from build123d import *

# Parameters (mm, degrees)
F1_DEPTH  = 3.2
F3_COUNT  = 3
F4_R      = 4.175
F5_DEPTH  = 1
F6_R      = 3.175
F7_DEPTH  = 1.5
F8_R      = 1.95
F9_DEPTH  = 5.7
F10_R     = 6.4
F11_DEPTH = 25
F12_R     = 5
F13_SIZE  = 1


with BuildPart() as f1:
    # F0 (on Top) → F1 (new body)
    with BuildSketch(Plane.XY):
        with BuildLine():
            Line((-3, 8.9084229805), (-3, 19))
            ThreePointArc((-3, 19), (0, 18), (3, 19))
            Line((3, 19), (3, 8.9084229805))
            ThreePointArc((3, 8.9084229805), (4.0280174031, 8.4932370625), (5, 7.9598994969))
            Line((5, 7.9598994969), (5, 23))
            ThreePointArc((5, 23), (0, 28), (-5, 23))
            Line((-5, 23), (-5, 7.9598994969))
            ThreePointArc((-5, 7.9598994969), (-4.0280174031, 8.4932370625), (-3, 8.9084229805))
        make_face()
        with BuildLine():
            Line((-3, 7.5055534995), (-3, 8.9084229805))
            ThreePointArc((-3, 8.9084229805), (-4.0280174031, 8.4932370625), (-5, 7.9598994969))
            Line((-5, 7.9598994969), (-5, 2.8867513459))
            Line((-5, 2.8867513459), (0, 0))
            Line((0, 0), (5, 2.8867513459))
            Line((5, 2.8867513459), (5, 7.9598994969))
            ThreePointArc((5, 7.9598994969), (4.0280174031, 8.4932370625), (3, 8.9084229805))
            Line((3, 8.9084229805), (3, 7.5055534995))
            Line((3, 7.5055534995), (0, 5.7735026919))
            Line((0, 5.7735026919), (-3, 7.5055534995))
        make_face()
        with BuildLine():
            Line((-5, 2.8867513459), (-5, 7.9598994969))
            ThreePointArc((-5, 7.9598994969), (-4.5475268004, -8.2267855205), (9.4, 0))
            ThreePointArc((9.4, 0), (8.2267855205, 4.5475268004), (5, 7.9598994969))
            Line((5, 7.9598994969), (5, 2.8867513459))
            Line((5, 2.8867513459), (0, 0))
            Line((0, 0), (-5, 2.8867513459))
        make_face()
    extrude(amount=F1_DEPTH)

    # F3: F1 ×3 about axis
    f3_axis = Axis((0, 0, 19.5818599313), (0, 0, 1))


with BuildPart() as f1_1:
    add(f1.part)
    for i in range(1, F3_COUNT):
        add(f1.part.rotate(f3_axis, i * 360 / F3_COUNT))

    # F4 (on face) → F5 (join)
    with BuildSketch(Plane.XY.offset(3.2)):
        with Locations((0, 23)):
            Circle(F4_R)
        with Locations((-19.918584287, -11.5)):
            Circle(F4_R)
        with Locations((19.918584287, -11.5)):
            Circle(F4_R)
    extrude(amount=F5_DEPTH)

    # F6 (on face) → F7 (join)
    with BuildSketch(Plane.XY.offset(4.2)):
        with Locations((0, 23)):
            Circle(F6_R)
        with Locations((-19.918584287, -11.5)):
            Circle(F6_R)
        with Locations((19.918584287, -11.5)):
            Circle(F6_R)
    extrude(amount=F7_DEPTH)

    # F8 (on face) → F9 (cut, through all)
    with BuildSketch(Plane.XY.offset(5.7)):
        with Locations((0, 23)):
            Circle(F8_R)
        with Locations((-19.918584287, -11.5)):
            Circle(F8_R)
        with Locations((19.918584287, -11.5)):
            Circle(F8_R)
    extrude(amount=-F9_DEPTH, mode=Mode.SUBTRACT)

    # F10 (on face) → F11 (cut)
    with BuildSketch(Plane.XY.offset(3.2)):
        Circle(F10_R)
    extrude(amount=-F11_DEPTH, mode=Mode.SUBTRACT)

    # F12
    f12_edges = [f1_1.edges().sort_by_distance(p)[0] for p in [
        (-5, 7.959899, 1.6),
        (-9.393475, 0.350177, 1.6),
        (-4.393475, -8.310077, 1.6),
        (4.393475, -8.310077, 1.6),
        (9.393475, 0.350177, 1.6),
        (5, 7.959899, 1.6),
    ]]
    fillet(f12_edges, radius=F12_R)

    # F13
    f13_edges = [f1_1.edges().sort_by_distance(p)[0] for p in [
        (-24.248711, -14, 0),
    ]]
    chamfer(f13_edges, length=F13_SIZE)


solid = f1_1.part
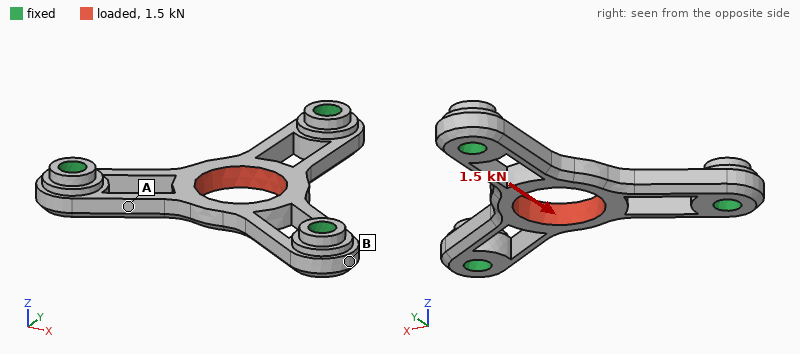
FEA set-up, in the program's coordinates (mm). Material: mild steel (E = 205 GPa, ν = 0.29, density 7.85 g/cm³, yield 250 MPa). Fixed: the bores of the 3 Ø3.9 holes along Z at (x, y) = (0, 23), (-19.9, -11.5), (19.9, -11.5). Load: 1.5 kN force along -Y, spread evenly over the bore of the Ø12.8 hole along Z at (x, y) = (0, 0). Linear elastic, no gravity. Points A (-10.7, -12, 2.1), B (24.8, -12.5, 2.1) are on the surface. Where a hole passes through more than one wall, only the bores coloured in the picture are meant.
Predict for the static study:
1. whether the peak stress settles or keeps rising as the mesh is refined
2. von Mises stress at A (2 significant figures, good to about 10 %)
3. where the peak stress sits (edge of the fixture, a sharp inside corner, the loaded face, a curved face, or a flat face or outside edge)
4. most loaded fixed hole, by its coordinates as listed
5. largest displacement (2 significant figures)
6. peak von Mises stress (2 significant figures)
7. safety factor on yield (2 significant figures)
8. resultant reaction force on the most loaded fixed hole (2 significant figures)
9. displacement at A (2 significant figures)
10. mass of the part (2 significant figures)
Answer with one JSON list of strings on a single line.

["settles", "85 MPa", "the loaded face", "(0, 23)", "17 µm", "150 MPa", "1.6", "960 N", "5.7 µm", "13 g"]
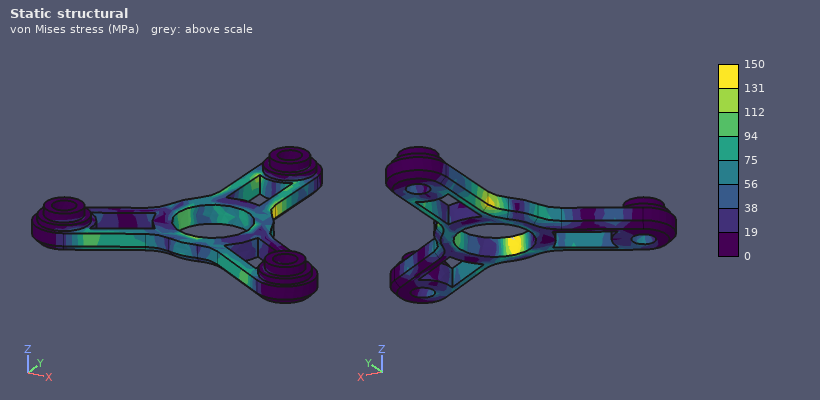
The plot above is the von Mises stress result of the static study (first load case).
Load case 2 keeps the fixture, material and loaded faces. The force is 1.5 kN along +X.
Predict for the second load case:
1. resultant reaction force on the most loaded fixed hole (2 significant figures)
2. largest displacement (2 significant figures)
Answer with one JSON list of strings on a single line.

["830 N", "15 µm"]
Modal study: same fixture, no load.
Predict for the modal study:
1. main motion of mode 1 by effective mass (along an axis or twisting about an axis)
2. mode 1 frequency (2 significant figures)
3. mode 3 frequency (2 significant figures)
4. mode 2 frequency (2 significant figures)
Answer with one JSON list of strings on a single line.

["along Z", "9200 Hz", "16 kHz", "16 kHz"]
